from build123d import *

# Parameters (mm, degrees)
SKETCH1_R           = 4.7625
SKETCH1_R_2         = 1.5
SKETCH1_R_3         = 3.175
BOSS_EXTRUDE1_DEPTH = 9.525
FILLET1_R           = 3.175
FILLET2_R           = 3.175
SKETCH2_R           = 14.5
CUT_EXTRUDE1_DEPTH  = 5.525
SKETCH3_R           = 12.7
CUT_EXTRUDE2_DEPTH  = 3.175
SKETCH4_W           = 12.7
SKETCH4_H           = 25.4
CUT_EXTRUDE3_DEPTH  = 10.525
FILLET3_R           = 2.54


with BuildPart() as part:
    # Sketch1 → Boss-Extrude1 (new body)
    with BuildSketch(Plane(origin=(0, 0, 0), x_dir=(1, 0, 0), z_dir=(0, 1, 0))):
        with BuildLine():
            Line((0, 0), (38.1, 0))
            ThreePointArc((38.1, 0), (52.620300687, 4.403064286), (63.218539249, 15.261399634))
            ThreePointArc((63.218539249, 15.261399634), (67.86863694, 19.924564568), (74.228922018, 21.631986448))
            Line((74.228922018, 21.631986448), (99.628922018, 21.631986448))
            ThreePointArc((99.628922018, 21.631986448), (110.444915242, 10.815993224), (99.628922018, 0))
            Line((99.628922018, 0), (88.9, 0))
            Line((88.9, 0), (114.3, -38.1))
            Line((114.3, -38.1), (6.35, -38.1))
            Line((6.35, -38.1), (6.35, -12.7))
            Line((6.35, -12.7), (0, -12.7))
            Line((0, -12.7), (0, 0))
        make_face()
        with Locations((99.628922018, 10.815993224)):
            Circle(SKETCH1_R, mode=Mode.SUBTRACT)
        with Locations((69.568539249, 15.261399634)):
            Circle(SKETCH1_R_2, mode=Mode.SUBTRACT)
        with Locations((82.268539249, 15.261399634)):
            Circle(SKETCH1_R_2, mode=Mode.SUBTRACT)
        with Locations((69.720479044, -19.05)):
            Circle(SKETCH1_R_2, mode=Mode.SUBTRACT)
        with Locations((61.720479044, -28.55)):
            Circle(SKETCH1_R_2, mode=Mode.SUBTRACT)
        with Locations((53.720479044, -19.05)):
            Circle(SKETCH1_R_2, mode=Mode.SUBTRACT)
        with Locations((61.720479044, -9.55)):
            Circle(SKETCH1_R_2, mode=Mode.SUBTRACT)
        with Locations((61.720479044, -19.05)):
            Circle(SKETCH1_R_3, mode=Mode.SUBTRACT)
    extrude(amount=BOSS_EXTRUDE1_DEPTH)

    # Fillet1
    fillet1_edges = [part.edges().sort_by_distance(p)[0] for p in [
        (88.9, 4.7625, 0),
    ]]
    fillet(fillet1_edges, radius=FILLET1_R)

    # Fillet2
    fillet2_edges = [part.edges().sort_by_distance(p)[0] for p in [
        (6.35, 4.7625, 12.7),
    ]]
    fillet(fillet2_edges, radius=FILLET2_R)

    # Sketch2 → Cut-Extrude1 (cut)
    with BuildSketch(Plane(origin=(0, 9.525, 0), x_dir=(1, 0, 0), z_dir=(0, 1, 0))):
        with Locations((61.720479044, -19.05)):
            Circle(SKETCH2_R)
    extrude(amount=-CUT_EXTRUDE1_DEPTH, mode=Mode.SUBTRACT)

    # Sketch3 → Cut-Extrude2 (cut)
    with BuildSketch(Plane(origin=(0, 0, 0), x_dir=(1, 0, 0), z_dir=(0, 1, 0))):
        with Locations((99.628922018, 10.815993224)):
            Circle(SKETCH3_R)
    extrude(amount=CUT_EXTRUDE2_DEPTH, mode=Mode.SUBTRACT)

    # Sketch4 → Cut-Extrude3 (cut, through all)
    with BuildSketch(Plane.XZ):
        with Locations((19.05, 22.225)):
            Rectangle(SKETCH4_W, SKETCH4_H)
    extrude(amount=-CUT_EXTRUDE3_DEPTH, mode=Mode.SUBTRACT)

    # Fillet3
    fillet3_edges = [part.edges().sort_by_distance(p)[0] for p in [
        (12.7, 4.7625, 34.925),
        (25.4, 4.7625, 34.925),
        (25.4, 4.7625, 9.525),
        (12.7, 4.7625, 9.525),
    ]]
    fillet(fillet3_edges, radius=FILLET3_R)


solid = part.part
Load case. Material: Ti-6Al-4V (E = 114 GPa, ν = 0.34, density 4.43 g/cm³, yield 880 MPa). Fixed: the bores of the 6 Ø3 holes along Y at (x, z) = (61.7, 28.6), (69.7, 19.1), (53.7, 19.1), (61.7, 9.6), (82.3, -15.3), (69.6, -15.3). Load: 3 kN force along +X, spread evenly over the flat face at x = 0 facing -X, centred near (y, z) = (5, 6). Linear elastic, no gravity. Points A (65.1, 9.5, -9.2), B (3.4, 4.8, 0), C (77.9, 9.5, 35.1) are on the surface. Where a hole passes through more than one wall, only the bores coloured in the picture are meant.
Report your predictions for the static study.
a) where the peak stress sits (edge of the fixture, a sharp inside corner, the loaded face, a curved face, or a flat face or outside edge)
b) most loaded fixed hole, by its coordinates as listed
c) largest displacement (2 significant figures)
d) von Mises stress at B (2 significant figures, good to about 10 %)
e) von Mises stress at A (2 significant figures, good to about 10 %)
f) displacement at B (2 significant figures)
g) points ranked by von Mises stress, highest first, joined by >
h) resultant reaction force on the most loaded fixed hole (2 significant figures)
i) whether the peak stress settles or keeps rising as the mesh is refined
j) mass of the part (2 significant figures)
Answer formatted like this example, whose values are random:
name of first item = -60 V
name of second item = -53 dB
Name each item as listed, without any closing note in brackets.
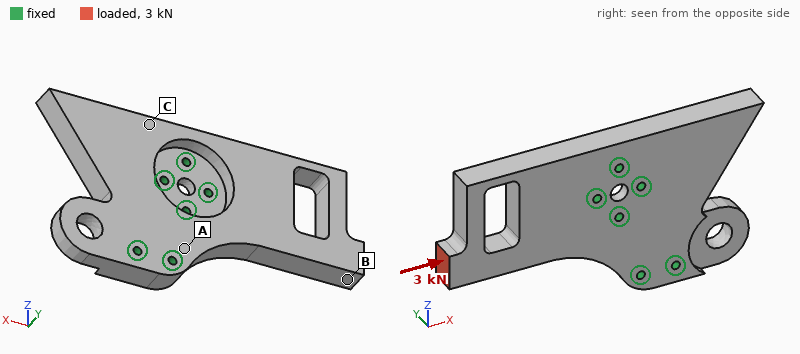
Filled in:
where the peak stress sits = edge of the fixture
most loaded fixed hole, by its coordinates as listed = (61.7, 9.6)
largest displacement = 32 µm
von Mises stress at B = 25 MPa
von Mises stress at A = 16 MPa
displacement at B = 29 µm
points ranked by von Mises stress, highest first, joined by > = B > A > C
resultant reaction force on the most loaded fixed hole = 1.0 kN
whether the peak stress settles or keeps rising as the mesh is refined = keeps rising
mass of the part = 160 g
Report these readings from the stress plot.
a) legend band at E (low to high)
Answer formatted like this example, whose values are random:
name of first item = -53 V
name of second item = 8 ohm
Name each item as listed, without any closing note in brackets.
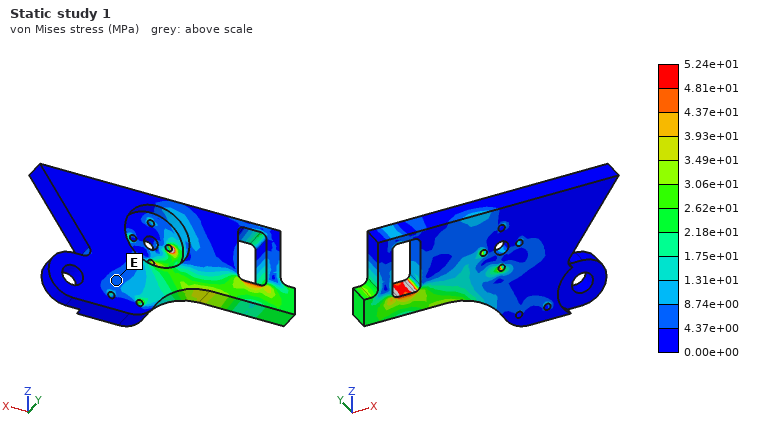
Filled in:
legend band at E = 4.37e+00 to 8.74e+00 MPa
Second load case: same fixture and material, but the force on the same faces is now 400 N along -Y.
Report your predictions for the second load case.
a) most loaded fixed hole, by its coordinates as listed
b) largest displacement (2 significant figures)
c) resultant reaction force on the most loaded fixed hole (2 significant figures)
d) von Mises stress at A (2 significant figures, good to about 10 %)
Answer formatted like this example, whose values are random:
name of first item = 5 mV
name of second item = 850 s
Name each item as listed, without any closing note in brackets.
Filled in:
most loaded fixed hole, by its coordinates as listed = (53.7, 19.1)
largest displacement = 0.20 mm
resultant reaction force on the most loaded fixed hole = 1.2 kN
von Mises stress at A = 23 MPa
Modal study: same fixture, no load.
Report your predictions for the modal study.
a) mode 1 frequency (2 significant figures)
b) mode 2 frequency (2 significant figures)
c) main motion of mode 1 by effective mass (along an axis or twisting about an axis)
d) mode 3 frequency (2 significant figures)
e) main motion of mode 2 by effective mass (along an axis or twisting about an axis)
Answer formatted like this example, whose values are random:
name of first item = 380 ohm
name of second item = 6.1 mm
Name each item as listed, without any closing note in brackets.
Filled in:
mode 1 frequency = 2100 Hz
mode 2 frequency = 3900 Hz
main motion of mode 1 by effective mass = along Y
mode 3 frequency = 5400 Hz
main motion of mode 2 by effective mass = along Y
